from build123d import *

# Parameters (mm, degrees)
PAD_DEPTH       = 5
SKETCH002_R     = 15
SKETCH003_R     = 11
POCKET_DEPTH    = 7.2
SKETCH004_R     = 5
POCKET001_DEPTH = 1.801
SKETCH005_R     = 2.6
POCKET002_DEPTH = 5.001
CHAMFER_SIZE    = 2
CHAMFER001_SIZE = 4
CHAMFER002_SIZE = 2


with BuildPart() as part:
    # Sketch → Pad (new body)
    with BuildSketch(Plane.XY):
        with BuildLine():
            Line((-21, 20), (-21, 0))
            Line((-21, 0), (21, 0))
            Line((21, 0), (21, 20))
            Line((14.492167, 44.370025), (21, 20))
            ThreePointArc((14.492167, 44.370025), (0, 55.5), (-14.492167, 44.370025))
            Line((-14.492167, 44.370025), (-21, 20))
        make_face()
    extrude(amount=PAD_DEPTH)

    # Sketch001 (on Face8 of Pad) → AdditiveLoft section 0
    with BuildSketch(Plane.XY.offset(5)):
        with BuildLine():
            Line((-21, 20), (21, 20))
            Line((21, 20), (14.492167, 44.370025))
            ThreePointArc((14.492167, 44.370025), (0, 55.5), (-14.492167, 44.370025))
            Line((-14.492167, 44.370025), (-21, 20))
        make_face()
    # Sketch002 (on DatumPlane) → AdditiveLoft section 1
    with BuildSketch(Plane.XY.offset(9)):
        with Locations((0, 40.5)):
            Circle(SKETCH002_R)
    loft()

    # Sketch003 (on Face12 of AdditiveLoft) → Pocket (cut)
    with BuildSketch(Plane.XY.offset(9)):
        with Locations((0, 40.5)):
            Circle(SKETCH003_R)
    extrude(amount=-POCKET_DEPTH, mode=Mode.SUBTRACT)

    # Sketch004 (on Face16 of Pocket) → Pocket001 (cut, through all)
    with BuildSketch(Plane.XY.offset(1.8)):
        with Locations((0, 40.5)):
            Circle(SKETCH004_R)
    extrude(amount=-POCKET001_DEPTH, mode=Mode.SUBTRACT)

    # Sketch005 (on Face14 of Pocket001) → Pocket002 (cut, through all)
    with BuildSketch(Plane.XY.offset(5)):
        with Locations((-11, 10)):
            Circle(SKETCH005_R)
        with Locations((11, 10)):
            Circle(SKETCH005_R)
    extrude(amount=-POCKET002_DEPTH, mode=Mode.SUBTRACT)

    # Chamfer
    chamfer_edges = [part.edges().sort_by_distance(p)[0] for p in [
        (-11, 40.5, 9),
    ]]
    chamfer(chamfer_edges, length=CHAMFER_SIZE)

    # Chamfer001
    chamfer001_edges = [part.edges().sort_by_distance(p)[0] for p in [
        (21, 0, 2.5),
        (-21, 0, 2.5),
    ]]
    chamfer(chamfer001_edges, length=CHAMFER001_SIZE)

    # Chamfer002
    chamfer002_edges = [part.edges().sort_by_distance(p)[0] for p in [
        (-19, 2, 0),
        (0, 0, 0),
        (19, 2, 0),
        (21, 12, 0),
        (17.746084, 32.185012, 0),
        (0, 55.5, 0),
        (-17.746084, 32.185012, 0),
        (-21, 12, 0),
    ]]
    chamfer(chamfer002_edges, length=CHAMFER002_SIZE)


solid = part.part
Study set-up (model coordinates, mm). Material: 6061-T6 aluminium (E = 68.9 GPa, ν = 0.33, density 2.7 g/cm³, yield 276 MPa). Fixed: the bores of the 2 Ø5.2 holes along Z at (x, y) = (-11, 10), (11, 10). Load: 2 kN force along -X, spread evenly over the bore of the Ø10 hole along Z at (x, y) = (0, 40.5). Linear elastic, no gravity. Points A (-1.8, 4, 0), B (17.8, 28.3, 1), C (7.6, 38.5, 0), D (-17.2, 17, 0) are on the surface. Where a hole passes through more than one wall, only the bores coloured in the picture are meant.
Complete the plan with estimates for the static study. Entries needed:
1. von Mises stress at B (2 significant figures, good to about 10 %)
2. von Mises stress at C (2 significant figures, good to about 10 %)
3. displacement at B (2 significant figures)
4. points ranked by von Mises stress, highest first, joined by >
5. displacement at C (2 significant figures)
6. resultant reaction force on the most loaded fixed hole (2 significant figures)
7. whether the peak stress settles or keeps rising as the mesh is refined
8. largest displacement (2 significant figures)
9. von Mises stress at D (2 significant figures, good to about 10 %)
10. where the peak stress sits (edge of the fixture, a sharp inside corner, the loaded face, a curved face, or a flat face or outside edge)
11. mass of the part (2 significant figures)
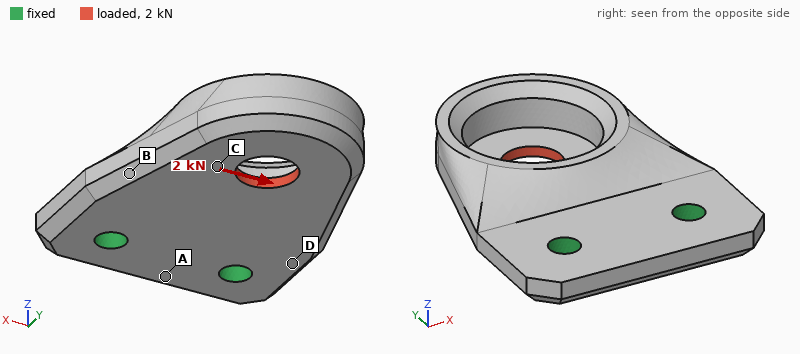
36 MPa
60 MPa
23 µm
C > B > D > A
34 µm
2.6 kN
keeps rising
51 µm
17 MPa
edge of the fixture
26 g
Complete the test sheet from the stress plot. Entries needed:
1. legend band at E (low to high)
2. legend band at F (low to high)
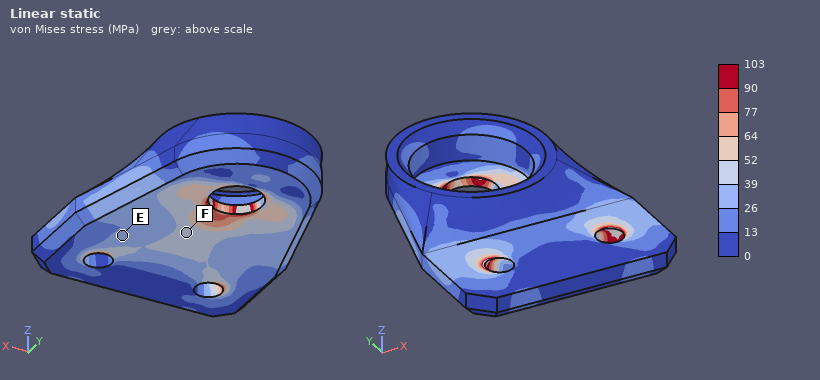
26 to 39 MPa
39 to 52 MPa
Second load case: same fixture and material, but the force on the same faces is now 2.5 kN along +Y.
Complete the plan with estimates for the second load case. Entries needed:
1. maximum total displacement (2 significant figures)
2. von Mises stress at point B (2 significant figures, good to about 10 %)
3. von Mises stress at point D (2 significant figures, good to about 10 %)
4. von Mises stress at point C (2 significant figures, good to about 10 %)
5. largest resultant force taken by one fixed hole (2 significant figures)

0.10 mm
23 MPa
30 MPa
47 MPa
1.3 kN
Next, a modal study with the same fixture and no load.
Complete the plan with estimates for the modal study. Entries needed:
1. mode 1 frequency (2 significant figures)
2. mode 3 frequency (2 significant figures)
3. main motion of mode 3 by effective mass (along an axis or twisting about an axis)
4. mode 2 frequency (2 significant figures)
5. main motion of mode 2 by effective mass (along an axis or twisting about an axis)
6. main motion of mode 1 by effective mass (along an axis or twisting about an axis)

2900 Hz
11 kHz
along X
8300 Hz
twisting about Y
along Z
